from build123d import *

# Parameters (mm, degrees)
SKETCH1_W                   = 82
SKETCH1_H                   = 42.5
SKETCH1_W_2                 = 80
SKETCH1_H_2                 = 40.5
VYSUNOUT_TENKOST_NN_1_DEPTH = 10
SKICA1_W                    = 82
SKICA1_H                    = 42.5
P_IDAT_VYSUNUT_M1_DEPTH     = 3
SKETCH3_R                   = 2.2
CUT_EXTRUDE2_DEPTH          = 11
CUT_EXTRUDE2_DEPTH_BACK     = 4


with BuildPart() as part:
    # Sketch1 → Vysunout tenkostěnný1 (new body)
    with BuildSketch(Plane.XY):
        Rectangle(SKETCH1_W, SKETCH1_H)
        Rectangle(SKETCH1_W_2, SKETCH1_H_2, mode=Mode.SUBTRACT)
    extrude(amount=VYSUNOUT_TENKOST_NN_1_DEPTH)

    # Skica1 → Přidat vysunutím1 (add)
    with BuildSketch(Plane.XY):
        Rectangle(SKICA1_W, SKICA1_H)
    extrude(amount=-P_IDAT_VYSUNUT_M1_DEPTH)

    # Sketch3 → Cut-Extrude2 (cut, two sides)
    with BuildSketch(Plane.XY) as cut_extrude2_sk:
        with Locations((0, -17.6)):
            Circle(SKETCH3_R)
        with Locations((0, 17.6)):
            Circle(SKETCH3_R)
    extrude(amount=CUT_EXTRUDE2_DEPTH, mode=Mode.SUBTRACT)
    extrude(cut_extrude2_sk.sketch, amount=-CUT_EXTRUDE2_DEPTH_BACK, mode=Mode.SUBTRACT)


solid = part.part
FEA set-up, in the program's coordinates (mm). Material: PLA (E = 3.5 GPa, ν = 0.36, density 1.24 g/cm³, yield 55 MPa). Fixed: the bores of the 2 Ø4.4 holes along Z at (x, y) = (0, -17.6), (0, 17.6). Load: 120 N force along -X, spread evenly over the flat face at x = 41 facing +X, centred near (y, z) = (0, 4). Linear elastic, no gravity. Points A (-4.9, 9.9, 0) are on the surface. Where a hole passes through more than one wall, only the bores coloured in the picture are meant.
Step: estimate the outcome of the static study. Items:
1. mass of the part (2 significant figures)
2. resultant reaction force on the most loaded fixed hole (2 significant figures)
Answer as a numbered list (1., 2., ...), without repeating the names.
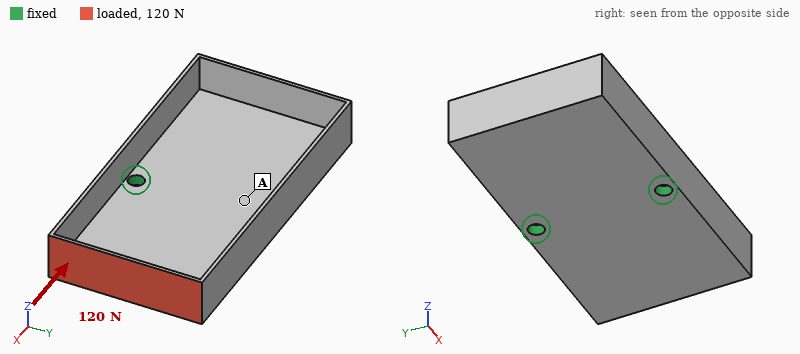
1. 16 g
2. 60 N
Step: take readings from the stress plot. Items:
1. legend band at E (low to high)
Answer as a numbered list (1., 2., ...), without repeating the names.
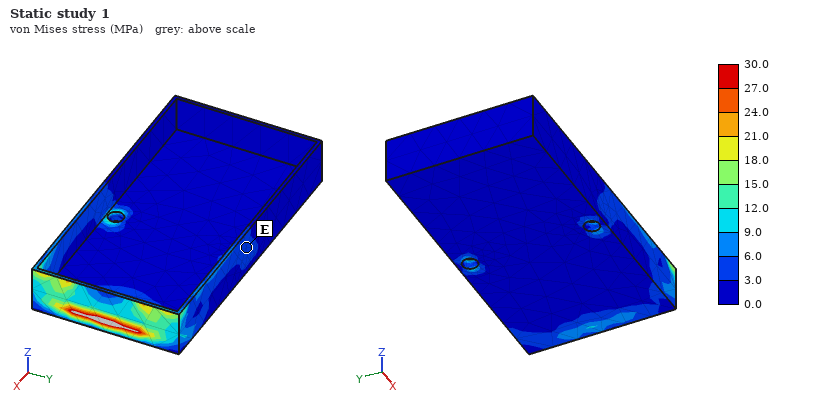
1. 3.0 to 6.0 MPa
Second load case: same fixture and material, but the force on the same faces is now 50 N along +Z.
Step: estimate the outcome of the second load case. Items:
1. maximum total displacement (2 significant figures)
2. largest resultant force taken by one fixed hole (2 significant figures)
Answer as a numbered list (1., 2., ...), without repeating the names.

1. 0.95 mm
2. 25 N
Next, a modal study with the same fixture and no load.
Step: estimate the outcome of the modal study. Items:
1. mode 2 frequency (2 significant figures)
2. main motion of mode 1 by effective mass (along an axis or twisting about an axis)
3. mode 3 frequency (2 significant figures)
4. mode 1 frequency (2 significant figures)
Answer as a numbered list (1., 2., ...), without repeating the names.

1. 1100 Hz
2. twisting about Y
3. 1100 Hz
4. 600 Hz
